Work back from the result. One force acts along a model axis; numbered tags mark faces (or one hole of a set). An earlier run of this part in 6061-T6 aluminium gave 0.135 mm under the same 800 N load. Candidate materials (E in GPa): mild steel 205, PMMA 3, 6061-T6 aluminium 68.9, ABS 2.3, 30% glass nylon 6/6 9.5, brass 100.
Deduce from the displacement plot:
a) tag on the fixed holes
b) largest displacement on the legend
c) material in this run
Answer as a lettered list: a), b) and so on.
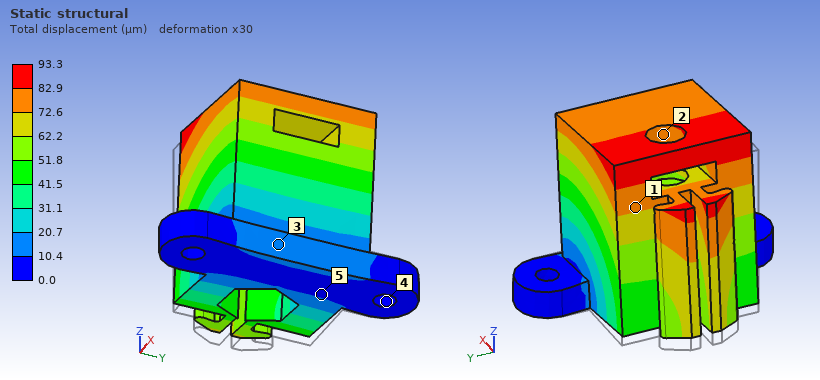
a) 4
b) 93.3 µm
c) brass
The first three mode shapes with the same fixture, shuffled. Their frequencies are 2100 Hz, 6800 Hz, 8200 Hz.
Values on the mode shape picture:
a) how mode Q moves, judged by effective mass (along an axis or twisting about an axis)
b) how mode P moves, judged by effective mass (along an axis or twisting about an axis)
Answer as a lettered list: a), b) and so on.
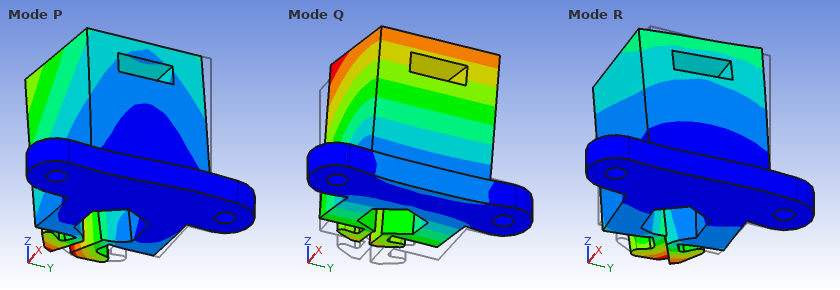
a) along X
b) along Y
